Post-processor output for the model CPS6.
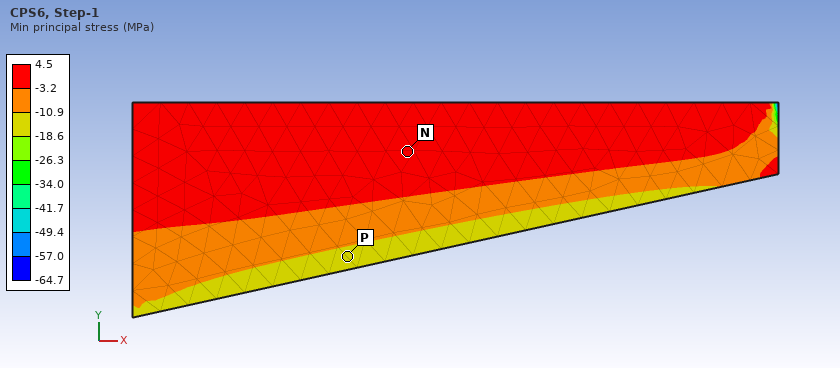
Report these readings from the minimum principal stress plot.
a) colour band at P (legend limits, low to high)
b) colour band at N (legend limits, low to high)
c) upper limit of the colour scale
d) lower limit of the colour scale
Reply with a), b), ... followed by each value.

a) -18.6 to -10.9 MPa
b) -3.2 to 4.5 MPa
c) 4.5 MPa
d) -64.7 MPa
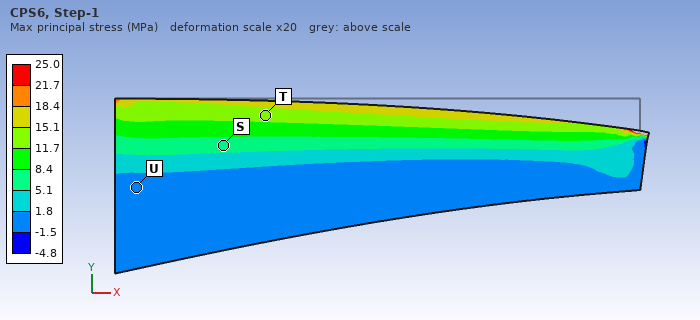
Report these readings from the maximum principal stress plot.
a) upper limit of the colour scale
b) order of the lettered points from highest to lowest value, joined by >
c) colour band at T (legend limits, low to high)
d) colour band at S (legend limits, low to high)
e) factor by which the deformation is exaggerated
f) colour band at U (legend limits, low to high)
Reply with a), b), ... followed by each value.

a) 25.0 MPa
b) T > S > U
c) 11.7 to 15.1 MPa
d) 5.1 to 8.4 MPa
e) 20
f) -1.5 to 1.8 MPa
